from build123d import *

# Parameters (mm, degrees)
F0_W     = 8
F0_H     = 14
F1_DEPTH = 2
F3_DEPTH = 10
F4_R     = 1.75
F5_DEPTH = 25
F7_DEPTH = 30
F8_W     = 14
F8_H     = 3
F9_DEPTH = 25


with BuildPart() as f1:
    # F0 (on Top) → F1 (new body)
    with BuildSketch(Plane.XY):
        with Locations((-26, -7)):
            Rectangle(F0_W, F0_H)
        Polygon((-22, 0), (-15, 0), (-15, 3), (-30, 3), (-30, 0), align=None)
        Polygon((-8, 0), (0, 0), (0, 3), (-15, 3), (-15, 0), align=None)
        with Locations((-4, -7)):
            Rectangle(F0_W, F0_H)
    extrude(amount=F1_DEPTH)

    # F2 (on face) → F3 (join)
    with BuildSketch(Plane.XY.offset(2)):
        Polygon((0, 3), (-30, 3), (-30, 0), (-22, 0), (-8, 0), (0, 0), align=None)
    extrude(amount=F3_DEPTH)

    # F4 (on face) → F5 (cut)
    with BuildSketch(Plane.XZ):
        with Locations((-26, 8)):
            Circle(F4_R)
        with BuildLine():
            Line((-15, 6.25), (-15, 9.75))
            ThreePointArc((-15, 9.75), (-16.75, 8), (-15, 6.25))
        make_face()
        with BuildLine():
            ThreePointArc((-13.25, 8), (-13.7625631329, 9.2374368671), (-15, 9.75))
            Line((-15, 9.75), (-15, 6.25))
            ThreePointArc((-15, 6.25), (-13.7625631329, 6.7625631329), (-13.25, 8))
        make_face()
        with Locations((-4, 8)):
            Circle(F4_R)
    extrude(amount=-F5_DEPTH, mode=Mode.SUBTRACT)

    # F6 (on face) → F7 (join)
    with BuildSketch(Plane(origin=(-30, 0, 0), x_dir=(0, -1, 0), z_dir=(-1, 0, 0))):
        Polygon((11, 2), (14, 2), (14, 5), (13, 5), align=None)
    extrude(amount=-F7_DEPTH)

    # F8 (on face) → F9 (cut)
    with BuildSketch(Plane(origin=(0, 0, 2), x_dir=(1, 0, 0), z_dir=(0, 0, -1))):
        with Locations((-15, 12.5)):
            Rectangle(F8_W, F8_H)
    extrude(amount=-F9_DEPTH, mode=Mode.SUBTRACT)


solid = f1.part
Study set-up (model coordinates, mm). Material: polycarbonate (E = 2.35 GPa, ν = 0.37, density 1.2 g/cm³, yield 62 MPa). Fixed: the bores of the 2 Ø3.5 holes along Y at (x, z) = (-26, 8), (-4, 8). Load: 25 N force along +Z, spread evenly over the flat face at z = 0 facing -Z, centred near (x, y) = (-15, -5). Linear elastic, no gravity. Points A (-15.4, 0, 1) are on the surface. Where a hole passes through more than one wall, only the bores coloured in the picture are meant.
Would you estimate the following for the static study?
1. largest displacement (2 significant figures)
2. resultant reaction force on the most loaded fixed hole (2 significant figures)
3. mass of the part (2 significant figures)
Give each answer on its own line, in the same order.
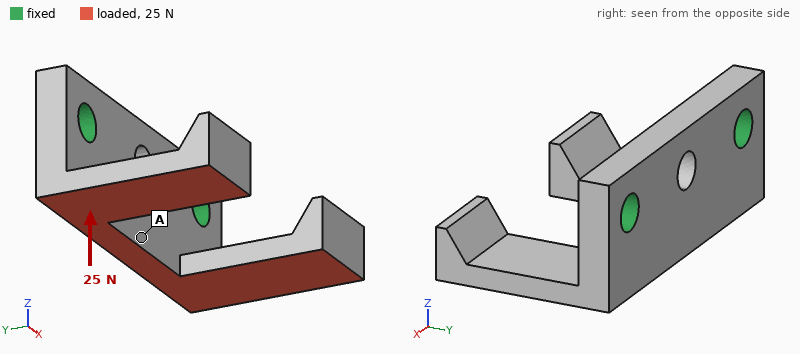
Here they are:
0.43 mm
13 N
1.8 g
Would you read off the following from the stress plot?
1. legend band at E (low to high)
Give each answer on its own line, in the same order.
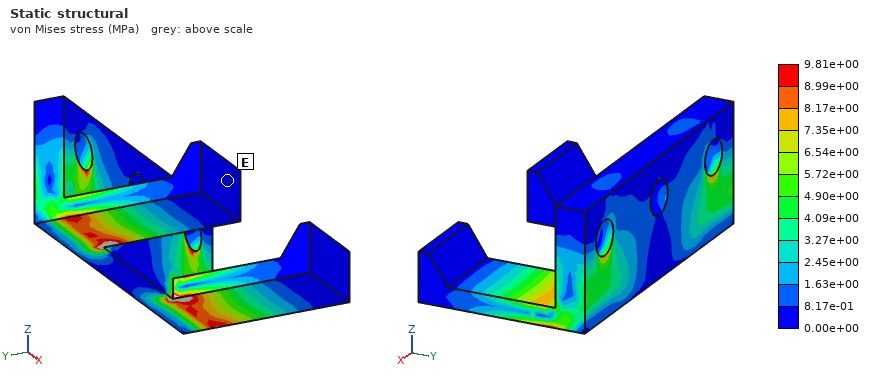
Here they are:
0.00e+00 to 8.17e-01 MPa
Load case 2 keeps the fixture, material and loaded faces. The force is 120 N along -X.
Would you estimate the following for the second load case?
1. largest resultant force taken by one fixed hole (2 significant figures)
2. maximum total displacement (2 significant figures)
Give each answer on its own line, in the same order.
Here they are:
71 N
0.43 mm
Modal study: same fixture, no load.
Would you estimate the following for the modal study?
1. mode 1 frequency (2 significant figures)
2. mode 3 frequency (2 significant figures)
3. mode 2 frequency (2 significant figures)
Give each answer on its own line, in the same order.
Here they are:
1400 Hz
2600 Hz
1400 Hz
